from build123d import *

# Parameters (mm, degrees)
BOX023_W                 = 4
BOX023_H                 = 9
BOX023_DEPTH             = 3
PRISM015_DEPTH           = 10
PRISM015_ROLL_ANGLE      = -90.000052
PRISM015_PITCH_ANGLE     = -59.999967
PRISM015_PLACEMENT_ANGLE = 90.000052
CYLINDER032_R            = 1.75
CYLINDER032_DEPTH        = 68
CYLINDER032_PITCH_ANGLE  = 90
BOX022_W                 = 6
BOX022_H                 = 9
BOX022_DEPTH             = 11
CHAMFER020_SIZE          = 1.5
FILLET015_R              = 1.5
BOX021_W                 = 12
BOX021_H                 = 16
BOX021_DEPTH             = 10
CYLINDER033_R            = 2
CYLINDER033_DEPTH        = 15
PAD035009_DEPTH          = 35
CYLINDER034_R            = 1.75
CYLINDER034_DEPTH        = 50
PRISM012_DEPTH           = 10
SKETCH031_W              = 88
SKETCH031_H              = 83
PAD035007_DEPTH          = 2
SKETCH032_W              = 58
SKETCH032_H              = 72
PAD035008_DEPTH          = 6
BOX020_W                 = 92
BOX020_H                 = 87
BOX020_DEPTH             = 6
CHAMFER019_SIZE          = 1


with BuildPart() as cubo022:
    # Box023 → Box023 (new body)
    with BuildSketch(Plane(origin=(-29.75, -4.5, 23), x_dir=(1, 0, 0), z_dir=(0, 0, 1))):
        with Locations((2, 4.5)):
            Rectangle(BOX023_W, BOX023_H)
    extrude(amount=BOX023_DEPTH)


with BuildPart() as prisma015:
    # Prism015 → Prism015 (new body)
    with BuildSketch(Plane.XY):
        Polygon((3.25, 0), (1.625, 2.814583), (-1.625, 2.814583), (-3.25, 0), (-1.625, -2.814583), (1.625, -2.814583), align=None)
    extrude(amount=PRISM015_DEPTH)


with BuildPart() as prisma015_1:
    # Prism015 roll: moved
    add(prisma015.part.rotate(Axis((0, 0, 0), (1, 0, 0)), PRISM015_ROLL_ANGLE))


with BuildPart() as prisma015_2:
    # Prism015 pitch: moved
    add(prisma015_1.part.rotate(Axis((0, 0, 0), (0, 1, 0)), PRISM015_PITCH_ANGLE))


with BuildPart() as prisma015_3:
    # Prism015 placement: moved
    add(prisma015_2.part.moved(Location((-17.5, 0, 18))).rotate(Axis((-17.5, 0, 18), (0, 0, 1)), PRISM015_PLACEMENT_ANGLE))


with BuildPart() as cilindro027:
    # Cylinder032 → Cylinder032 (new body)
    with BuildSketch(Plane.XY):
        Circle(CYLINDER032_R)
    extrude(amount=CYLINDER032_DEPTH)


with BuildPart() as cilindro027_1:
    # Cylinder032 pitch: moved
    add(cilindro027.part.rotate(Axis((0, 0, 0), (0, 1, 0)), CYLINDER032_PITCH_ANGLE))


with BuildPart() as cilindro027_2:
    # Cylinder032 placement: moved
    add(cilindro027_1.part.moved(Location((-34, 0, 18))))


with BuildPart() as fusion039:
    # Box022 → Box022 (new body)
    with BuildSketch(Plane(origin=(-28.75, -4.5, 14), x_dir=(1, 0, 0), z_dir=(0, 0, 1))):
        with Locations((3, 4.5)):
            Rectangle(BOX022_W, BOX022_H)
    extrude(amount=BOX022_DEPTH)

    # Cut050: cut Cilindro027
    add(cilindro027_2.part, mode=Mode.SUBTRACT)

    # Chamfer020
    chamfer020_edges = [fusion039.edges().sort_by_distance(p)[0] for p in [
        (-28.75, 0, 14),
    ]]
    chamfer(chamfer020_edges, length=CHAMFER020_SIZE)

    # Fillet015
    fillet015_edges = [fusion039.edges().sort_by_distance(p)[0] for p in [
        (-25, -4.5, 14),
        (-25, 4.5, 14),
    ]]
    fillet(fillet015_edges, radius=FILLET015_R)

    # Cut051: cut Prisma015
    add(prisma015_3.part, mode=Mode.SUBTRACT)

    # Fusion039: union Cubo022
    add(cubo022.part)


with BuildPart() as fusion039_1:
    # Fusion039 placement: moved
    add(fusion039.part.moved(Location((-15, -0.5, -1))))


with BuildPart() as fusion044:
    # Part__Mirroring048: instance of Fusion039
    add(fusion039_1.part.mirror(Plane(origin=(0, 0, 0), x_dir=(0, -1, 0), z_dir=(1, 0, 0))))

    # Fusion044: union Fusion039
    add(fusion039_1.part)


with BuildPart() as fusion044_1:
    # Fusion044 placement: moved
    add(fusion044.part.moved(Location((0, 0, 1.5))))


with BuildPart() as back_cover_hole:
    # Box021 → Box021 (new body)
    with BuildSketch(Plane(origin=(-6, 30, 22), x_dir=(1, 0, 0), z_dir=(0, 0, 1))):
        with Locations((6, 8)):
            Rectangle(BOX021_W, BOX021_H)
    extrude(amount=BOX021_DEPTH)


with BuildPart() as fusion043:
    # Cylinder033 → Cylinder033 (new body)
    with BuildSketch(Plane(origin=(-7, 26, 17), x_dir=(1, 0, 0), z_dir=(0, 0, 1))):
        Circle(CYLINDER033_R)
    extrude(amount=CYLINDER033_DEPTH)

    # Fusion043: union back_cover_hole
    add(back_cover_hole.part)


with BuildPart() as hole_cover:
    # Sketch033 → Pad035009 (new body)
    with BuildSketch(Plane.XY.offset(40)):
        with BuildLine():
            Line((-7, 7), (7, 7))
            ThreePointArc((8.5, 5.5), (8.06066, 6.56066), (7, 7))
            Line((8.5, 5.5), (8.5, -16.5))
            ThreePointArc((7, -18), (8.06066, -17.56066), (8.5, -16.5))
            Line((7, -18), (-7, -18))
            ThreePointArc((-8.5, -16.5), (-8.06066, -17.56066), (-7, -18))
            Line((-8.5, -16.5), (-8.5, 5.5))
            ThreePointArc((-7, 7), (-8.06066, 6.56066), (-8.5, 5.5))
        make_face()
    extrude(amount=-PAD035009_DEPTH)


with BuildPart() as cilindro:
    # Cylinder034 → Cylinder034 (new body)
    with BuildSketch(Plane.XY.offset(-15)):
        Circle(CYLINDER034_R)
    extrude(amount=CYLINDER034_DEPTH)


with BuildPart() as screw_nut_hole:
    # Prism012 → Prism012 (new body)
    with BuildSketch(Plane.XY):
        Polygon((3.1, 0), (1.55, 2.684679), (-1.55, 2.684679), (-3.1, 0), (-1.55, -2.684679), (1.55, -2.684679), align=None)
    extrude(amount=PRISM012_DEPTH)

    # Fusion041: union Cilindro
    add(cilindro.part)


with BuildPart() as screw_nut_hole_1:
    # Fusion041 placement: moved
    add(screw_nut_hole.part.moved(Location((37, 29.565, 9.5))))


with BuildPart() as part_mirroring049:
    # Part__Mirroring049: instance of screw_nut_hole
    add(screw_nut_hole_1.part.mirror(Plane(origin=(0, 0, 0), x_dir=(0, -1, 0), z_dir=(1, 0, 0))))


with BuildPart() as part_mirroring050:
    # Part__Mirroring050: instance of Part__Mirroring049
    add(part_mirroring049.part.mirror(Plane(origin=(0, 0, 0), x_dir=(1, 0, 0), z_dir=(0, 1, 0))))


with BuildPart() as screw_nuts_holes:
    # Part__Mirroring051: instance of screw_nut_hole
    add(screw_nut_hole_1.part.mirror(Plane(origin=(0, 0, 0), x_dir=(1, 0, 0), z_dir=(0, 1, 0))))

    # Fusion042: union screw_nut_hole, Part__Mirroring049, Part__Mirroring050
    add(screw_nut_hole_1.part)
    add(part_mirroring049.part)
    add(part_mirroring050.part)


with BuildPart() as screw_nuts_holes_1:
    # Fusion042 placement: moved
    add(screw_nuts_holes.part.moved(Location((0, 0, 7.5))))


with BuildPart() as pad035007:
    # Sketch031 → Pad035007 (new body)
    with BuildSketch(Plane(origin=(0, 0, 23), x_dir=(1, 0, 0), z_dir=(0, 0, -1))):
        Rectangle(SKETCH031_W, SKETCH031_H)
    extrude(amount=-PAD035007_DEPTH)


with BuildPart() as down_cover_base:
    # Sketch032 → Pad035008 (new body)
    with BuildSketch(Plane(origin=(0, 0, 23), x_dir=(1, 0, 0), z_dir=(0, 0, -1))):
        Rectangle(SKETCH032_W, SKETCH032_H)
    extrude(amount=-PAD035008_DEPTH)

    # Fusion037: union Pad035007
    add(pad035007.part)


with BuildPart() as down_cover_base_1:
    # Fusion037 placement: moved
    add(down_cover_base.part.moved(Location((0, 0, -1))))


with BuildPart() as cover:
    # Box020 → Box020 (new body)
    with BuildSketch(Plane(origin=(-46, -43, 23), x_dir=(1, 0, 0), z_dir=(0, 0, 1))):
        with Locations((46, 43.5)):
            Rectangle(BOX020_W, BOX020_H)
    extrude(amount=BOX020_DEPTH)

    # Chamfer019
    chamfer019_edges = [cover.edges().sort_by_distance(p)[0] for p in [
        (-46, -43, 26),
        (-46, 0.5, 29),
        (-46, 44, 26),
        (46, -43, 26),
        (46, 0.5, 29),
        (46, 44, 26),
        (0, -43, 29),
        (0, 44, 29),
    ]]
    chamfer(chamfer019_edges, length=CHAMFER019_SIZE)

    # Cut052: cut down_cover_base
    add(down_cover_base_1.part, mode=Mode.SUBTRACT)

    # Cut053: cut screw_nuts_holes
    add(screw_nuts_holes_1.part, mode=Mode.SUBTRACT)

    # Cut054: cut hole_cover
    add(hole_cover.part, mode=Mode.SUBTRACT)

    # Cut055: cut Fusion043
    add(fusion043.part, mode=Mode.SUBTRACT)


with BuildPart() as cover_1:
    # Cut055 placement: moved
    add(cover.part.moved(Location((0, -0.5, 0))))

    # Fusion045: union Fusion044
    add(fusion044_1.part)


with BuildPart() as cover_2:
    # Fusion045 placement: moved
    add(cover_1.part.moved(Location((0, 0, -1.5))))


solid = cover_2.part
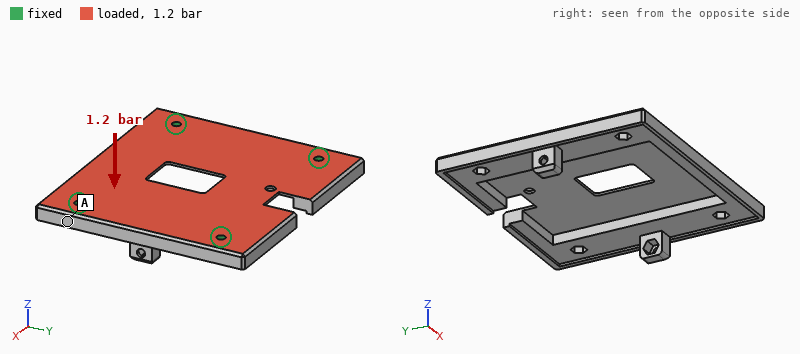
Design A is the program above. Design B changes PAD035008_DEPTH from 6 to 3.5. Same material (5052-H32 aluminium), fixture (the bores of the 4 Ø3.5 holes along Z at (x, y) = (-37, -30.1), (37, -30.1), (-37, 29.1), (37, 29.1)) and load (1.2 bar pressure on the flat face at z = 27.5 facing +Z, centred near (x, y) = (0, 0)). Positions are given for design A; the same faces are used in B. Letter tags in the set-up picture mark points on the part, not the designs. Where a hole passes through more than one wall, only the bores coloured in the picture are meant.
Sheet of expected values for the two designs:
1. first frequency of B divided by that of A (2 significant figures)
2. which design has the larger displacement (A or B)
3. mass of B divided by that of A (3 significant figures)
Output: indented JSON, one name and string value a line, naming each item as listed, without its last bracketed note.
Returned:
{
  "first frequency of B divided by that of A": "1.2",
  "which design has the larger displacement": "A",
  "mass of B divided by that of A": "1.40"
}
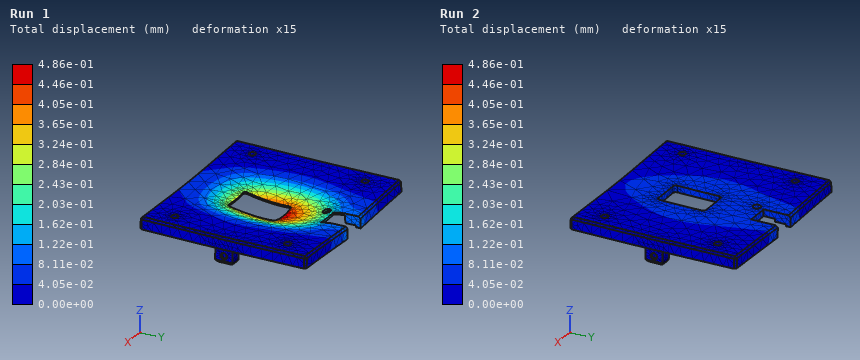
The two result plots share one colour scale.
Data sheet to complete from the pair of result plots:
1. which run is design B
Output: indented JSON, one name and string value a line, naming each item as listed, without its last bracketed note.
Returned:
{
  "which run is design B": "Run 2"
}
